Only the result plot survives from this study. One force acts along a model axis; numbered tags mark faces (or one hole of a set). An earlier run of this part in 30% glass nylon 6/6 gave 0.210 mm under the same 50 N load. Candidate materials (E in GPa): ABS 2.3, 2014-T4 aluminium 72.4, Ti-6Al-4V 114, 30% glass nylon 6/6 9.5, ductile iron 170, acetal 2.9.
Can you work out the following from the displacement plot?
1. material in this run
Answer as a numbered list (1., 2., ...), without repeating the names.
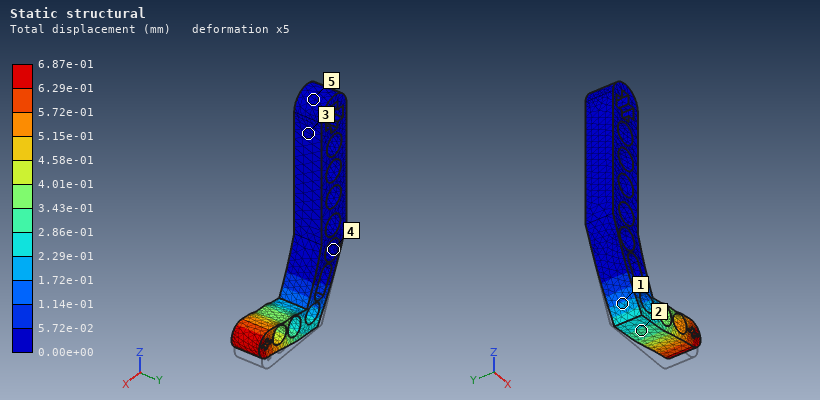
1. acetal
